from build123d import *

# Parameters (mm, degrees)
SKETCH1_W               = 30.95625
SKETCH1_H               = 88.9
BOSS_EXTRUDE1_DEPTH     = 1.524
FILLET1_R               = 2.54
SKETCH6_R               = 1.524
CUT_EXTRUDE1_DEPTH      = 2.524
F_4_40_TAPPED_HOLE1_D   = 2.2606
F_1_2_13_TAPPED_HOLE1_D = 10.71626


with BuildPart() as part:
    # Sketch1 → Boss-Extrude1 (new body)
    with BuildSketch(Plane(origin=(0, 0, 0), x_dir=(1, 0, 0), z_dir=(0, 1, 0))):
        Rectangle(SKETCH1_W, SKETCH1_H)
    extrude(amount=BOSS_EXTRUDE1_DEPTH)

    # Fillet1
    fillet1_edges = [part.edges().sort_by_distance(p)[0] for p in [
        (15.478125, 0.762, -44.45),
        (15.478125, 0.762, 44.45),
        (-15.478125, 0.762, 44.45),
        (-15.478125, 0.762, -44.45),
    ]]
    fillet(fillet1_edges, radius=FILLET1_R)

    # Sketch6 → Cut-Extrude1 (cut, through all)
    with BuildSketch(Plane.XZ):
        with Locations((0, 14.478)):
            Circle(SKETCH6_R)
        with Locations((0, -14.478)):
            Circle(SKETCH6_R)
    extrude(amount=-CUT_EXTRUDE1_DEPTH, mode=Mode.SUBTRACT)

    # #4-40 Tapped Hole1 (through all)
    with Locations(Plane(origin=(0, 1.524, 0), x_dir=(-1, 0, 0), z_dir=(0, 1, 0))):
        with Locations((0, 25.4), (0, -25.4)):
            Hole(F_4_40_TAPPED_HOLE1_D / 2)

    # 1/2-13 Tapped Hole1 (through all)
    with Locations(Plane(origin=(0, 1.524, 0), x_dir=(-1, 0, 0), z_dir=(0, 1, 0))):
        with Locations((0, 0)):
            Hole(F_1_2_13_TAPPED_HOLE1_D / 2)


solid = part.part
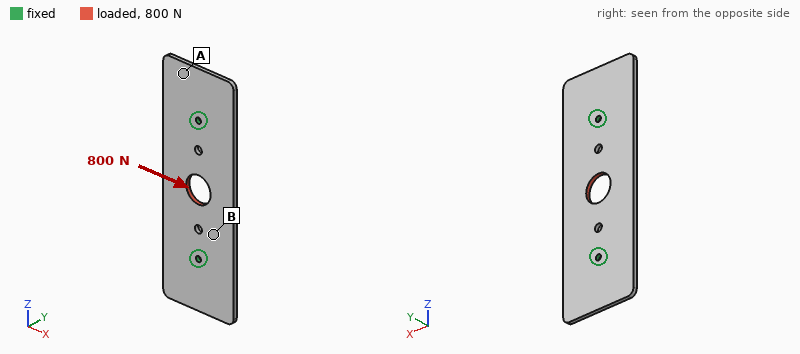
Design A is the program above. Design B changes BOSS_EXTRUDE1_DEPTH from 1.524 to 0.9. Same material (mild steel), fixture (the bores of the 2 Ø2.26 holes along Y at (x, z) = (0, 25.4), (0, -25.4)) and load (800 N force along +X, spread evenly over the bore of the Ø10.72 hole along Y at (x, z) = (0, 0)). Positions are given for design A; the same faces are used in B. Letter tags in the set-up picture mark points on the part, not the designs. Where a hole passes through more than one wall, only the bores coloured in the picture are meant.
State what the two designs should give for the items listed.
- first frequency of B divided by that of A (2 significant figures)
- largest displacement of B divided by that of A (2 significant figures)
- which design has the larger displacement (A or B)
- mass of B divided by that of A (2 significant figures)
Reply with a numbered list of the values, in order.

1. 0.61
2. 1.7
3. B
4. 0.59
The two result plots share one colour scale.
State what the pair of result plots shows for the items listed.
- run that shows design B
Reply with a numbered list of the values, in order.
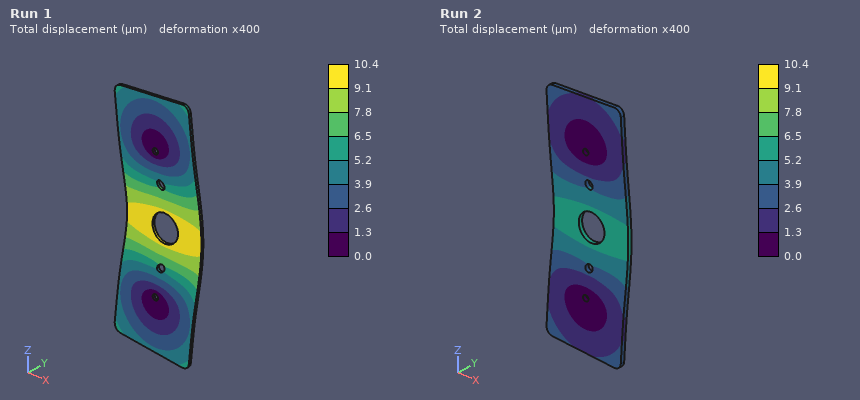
1. Run 1
